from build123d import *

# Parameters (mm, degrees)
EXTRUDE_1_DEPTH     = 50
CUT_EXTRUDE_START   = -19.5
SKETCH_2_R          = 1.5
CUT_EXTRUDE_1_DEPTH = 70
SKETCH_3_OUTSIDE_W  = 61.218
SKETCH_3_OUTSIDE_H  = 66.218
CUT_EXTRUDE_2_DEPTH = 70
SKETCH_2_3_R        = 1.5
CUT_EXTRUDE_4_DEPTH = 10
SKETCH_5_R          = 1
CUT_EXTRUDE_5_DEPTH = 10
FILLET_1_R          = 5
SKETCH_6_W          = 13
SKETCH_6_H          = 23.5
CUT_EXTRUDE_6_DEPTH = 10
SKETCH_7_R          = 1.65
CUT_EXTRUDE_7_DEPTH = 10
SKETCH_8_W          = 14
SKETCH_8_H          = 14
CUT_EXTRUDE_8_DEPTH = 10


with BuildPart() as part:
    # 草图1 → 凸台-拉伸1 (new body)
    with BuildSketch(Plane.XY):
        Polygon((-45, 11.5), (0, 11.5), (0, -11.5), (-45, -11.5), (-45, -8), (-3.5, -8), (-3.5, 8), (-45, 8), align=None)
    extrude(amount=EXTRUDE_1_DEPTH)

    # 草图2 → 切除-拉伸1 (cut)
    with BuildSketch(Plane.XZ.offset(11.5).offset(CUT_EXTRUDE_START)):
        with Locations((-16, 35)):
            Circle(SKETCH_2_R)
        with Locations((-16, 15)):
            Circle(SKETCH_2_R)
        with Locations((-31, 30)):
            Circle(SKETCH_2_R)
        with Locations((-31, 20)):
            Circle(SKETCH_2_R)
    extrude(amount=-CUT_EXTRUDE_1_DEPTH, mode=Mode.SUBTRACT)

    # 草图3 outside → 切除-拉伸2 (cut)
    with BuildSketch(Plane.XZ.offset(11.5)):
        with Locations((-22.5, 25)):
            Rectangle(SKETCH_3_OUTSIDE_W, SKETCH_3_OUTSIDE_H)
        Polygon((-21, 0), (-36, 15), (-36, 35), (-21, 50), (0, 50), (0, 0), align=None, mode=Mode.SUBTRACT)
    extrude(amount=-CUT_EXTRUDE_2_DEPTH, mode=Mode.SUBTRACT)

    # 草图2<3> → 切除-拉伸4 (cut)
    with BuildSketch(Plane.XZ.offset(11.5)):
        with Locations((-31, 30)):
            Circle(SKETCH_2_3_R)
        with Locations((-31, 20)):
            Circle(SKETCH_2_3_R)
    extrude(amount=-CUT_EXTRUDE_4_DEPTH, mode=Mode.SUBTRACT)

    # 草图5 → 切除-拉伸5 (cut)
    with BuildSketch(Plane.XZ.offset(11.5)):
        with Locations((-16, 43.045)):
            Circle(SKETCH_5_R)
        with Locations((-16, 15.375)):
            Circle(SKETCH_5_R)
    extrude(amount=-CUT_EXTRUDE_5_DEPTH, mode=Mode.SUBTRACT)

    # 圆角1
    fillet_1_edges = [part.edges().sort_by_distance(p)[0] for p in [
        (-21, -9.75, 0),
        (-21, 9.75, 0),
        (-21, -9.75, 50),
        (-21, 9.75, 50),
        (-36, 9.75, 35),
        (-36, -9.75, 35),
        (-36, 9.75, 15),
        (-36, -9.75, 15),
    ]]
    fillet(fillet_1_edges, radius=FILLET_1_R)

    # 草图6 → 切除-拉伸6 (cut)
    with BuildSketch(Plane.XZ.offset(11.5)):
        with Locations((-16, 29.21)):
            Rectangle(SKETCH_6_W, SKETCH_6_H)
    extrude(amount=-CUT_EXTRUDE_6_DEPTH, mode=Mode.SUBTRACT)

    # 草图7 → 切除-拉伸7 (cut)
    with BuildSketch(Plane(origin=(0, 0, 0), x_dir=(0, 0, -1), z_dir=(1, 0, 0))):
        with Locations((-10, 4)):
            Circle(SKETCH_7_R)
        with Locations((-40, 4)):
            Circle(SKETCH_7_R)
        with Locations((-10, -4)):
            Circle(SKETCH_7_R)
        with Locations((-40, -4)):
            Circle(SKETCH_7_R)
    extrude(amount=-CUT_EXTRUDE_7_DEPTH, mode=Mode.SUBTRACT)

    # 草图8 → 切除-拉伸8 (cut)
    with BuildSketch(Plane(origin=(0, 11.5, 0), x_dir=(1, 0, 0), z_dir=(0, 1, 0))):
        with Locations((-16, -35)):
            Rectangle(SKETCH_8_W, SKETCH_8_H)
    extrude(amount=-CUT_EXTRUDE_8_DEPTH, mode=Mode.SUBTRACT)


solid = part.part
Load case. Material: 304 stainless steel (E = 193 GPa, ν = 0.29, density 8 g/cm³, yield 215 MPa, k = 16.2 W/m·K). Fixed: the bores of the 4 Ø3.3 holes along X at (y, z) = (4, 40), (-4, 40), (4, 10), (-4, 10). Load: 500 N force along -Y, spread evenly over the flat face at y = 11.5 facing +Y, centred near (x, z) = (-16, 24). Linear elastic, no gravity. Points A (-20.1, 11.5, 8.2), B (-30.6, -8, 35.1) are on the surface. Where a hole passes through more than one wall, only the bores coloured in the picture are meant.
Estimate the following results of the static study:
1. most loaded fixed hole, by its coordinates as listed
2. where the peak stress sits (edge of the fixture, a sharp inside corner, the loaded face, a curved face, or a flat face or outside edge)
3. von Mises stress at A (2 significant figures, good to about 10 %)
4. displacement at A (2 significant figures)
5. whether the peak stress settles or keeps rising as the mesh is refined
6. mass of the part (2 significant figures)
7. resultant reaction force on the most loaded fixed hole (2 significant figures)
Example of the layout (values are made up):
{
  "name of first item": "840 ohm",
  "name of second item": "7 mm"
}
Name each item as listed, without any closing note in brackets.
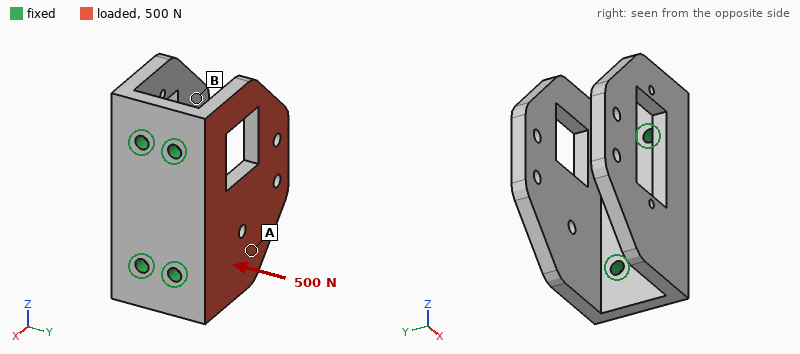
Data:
{
  "most loaded fixed hole, by its coordinates as listed": "(4, 10)",
  "where the peak stress sits": "edge of the fixture",
  "von Mises stress at A": "21 MPa",
  "displacement at A": "0.049 mm",
  "whether the peak stress settles or keeps rising as the mesh is refined": "keeps rising",
  "mass of the part": "94 g",
  "resultant reaction force on the most loaded fixed hole": "280 N"
}
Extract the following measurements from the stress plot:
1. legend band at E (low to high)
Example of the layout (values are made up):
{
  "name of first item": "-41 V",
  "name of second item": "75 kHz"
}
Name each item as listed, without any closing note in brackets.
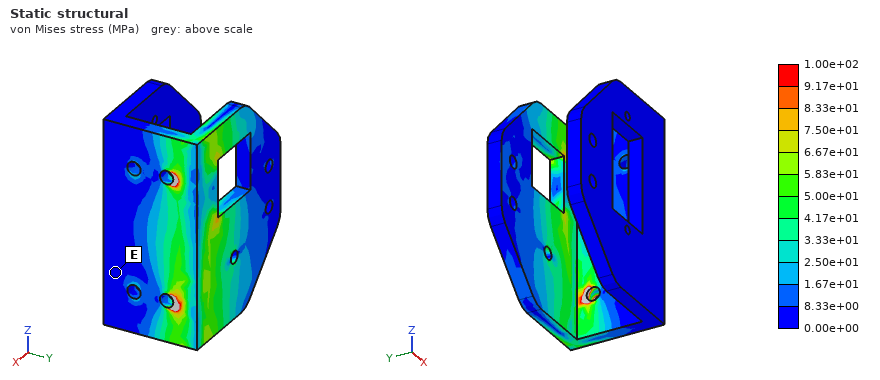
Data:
{
  "legend band at E": "0.00e+00 to 8.33e+00 MPa"
}
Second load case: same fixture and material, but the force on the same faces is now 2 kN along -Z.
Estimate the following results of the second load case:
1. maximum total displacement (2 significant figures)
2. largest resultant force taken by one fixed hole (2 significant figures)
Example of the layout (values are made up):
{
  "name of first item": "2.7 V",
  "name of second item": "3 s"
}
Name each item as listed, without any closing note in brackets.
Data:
{
  "maximum total displacement": "21 µm",
  "largest resultant force taken by one fixed hole": "1.3 kN"
}
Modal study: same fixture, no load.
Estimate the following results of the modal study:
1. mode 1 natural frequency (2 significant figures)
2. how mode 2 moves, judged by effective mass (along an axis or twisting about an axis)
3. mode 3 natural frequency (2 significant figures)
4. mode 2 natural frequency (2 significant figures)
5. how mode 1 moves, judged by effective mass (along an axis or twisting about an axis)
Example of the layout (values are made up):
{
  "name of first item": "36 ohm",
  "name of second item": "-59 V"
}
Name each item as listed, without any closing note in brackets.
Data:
{
  "mode 1 natural frequency": "2000 Hz",
  "how mode 2 moves, judged by effective mass": "along Y",
  "mode 3 natural frequency": "4900 Hz",
  "mode 2 natural frequency": "2200 Hz",
  "how mode 1 moves, judged by effective mass": "along Y"
}
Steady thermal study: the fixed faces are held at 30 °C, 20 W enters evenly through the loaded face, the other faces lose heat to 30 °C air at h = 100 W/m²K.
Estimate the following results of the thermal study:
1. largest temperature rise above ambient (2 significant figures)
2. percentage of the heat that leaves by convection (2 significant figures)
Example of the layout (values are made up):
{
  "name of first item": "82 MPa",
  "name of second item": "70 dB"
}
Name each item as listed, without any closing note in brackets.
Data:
{
  "largest temperature rise above ambient": "70 K",
  "percentage of the heat that leaves by convection": "60 %"
}
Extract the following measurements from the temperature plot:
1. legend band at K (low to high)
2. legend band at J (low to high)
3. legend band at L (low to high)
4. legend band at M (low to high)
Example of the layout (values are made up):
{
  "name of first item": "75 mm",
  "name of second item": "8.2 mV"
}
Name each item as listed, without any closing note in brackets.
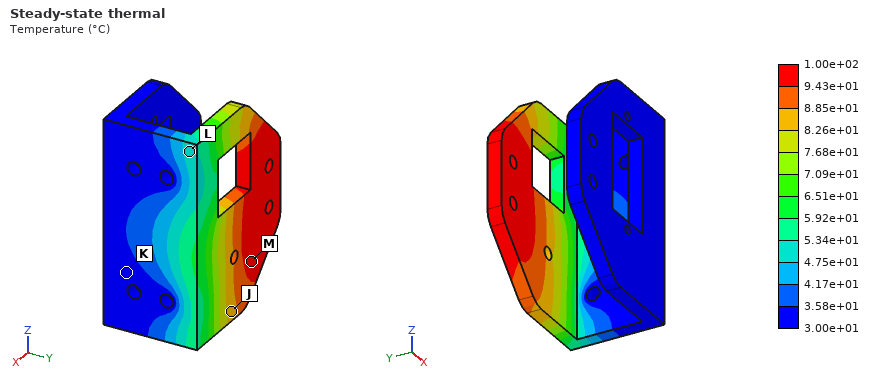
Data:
{
  "legend band at K": "3.00e+01 to 3.58e+01 °C",
  "legend band at J": "8.26e+01 to 8.85e+01 °C",
  "legend band at L": "4.75e+01 to 5.34e+01 °C",
  "legend band at M": "9.43e+01 to 1.00e+02 °C"
}
